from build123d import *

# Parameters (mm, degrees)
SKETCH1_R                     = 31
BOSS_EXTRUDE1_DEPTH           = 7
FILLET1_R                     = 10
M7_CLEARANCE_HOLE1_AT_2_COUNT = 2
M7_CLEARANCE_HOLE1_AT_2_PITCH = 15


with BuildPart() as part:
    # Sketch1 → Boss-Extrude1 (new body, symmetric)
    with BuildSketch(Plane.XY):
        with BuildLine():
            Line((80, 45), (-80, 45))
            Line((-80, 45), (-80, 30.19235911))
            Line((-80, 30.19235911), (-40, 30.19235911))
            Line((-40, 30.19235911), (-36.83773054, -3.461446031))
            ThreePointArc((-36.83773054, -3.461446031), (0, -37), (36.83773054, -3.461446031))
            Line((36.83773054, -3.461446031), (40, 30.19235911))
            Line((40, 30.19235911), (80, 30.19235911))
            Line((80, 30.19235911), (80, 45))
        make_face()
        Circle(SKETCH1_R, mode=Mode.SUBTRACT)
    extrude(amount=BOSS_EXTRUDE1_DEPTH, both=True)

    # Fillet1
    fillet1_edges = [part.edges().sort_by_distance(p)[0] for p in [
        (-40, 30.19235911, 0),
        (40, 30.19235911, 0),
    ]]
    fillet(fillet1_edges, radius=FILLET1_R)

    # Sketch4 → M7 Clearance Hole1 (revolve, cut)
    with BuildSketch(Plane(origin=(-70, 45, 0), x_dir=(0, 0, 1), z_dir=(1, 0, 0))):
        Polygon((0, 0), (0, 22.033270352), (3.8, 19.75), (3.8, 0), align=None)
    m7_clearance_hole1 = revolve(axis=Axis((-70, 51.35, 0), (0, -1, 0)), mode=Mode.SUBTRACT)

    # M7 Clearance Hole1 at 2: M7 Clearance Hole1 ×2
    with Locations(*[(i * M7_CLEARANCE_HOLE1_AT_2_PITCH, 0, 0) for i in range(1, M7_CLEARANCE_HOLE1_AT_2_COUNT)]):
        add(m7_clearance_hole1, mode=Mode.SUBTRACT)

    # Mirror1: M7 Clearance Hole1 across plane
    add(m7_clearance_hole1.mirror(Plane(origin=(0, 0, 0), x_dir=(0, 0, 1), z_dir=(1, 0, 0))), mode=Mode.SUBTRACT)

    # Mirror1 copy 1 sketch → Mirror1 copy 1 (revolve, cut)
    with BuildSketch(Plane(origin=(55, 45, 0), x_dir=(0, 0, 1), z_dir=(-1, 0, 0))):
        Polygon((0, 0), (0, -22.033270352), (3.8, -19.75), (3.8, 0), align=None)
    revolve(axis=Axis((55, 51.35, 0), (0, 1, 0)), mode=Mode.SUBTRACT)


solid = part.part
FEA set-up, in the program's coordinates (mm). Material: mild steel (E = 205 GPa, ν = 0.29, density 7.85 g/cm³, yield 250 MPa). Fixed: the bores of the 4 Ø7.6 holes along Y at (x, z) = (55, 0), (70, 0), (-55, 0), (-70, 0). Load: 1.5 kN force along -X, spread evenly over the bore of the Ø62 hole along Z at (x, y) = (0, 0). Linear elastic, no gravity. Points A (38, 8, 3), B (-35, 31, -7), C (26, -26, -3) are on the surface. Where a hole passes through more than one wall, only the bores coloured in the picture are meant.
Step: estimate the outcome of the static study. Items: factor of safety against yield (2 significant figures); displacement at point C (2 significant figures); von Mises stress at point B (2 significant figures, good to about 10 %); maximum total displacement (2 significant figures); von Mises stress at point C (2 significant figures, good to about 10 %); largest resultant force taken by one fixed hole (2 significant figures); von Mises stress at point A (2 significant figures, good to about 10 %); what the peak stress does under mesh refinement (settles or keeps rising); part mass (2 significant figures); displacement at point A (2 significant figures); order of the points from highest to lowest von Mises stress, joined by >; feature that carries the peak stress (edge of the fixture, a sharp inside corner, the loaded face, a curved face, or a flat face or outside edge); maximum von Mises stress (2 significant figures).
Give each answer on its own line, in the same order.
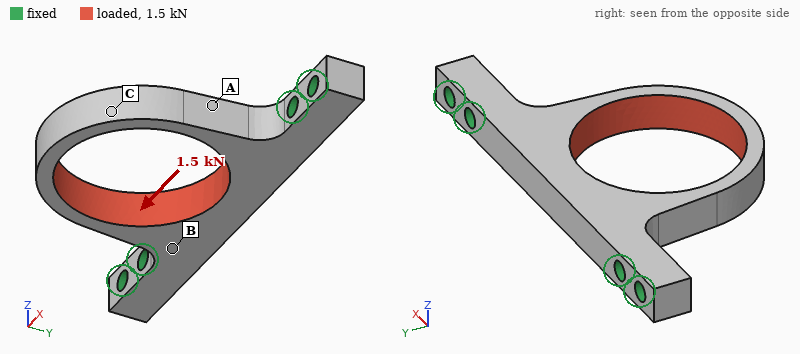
6.4
35 µm
5.7 MPa
36 µm
29 MPa
910 N
38 MPa
settles
400 g
6.6 µm
A > C > B
the loaded face
39 MPa
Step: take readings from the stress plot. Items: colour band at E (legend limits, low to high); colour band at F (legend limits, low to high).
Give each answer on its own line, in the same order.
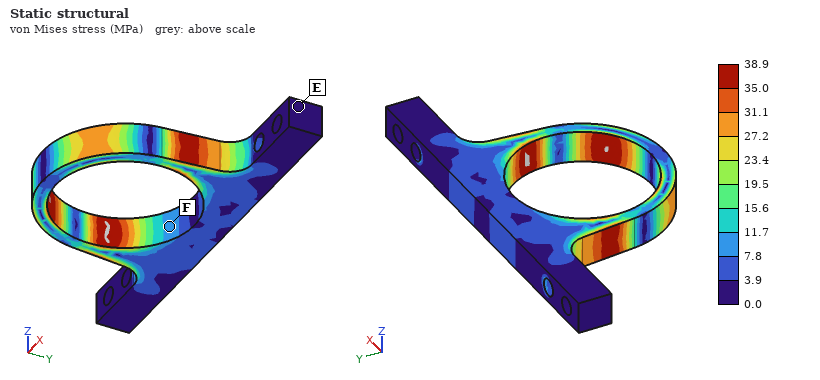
0.0 to 3.9 MPa
7.8 to 11.7 MPa
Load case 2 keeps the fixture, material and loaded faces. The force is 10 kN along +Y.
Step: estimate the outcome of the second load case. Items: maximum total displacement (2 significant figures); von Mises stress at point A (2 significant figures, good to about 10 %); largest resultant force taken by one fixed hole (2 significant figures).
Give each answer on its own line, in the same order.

35 µm
82 MPa
5.2 kN
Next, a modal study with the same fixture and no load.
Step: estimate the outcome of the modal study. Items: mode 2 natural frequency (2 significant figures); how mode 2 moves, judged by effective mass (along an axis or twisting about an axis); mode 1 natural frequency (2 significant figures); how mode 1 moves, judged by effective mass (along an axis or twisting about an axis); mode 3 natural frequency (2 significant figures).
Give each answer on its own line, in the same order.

3000 Hz
along X
1600 Hz
along Z
4000 Hz
